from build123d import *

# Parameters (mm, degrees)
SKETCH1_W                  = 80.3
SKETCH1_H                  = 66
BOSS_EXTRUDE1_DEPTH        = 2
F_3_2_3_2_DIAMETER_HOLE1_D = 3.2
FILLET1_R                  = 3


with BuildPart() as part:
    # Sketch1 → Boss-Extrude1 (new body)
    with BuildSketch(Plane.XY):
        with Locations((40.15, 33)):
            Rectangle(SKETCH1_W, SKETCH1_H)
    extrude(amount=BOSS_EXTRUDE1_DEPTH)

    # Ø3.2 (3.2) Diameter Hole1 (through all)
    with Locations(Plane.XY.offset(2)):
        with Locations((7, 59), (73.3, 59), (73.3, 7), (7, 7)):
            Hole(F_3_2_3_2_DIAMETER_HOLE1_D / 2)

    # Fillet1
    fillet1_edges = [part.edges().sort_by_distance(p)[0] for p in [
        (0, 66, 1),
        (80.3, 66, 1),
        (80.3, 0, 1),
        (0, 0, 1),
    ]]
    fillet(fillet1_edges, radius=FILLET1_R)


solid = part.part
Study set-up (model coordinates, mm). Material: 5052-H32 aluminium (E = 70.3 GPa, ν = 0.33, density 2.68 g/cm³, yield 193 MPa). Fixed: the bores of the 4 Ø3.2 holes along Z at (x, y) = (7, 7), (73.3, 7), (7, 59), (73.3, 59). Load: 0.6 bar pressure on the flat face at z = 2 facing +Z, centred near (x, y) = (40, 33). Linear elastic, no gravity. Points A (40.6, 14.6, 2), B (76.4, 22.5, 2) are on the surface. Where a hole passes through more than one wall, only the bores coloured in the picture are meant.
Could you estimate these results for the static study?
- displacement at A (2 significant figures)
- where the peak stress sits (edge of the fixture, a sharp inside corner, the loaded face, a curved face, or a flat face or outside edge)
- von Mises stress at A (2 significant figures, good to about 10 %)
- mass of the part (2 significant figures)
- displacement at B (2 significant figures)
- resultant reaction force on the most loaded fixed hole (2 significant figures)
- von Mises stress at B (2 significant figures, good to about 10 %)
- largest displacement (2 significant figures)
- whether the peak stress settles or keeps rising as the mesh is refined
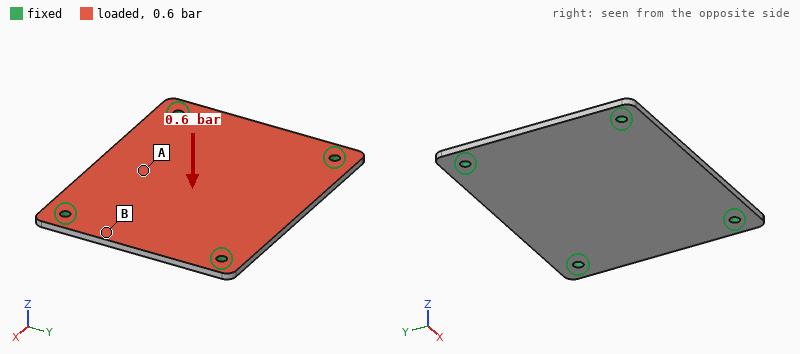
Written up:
0.093 mm
edge of the fixture
18 MPa
28 g
0.018 mm
79 N
8.1 MPa
0.11 mm
keeps rising
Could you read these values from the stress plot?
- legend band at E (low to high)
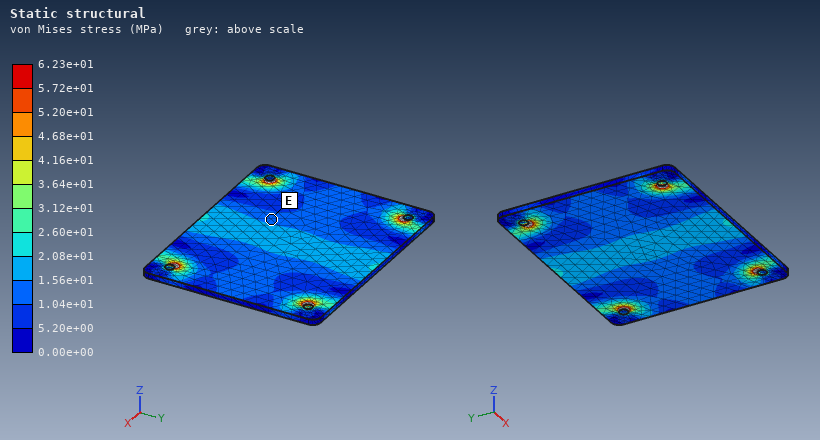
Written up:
1.04e+01 to 1.56e+01 MPa
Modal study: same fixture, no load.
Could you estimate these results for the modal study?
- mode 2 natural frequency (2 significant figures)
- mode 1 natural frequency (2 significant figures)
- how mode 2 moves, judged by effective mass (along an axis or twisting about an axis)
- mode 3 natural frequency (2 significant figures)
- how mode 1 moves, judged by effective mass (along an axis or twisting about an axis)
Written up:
2900 Hz
1900 Hz
twisting about X
3800 Hz
along Z
